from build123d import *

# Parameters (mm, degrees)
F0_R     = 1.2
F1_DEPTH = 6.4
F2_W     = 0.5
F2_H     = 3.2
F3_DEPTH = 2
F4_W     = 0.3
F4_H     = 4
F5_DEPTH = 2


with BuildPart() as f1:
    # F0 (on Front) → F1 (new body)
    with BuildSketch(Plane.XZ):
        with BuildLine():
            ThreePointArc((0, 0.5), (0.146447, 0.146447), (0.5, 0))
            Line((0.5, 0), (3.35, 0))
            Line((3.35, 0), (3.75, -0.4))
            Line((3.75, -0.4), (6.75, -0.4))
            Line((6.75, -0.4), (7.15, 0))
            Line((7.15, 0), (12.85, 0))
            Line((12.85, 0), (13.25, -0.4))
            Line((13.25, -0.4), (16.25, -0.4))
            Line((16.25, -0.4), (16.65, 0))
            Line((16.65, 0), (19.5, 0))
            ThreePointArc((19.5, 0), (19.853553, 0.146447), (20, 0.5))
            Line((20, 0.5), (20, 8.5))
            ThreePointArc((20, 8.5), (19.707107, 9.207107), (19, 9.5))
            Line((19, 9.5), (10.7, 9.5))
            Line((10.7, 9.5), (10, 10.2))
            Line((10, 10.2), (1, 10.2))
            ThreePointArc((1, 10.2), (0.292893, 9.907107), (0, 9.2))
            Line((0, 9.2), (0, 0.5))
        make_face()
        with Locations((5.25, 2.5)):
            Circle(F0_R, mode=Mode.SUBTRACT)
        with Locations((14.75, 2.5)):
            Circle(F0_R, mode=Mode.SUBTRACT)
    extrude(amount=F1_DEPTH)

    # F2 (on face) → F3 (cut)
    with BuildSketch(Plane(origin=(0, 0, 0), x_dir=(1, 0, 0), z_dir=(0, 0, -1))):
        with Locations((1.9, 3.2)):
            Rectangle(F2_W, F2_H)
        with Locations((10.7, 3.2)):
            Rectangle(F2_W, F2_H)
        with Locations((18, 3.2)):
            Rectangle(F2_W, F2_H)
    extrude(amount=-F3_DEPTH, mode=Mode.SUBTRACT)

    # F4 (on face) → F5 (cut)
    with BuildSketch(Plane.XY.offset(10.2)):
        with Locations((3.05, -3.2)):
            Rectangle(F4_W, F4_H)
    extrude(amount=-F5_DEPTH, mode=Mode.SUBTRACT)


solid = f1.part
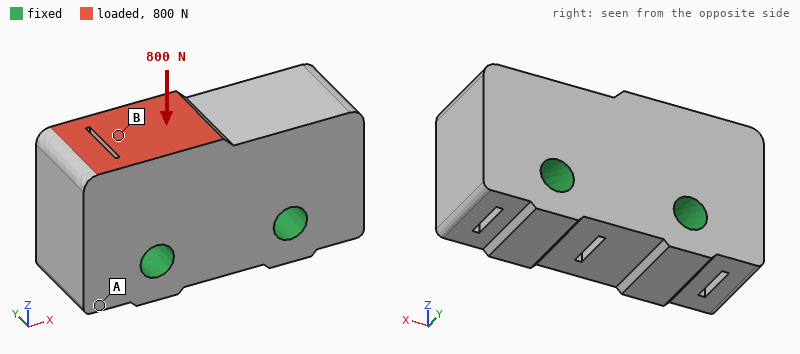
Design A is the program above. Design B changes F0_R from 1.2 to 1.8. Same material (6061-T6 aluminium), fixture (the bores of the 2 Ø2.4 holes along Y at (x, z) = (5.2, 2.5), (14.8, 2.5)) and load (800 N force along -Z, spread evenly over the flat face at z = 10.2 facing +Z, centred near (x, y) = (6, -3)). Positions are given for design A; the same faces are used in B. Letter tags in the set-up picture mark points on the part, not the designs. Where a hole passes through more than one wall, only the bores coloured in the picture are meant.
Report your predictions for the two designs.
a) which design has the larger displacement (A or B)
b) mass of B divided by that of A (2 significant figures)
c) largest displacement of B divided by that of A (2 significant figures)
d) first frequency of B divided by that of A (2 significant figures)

A
0.94
0.80
1.2
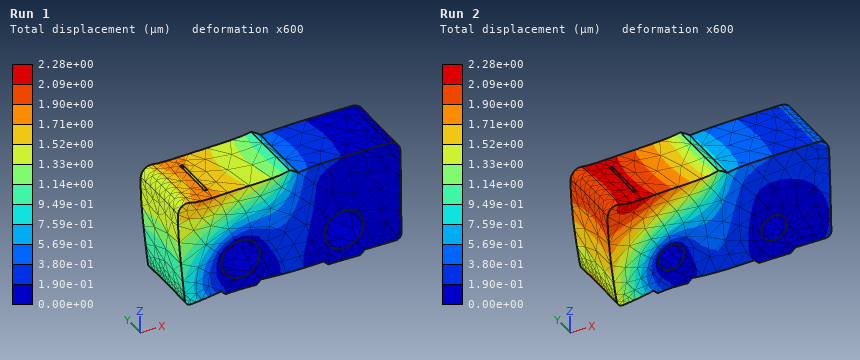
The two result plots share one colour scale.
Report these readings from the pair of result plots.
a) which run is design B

Run 1
